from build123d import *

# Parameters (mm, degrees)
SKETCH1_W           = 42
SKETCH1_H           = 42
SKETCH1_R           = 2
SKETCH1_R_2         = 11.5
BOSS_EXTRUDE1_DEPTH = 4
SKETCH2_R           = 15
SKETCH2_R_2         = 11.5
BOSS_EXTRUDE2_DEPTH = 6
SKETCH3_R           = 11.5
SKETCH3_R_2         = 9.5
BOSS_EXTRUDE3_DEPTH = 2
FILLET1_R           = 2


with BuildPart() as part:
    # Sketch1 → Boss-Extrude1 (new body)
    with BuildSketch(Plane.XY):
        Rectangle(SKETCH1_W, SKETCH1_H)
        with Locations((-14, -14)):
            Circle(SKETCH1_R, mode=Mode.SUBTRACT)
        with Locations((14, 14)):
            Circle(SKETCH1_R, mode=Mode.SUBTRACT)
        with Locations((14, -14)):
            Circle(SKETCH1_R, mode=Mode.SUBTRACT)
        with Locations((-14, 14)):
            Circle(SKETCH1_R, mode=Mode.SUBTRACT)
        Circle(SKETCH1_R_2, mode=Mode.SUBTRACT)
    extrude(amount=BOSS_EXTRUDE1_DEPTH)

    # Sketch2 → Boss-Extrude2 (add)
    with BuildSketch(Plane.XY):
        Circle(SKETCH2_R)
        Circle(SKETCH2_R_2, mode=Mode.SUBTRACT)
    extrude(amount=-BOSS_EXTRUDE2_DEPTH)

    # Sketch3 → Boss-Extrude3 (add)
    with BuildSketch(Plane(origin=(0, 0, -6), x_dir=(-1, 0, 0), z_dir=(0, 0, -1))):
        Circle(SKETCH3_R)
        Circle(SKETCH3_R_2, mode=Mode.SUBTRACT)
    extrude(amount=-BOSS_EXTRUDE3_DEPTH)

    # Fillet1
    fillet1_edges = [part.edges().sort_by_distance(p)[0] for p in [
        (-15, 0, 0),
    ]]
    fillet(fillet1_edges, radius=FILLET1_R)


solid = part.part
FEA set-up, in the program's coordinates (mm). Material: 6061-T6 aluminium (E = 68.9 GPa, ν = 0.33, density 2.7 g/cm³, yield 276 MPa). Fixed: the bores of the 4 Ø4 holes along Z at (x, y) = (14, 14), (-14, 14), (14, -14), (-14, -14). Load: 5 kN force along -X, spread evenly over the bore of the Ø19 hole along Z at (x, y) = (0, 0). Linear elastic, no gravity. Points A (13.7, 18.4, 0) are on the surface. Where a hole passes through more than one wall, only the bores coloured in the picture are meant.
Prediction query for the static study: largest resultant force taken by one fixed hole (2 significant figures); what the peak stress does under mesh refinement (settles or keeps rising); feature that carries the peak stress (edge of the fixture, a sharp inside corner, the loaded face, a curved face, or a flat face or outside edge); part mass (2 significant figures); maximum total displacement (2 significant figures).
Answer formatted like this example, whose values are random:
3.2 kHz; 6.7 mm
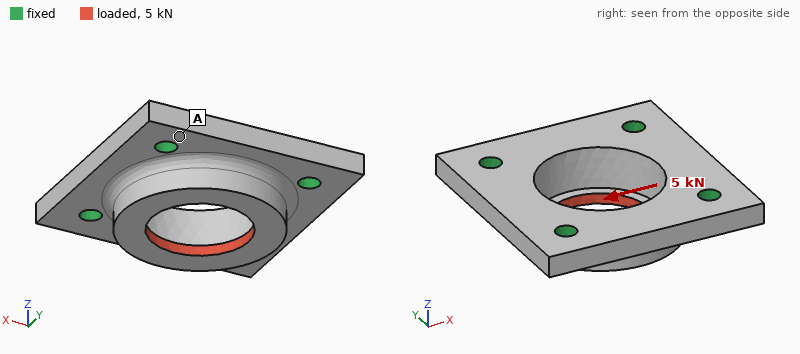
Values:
1.4 kN; keeps rising; edge of the fixture; 20 g; 28 µm
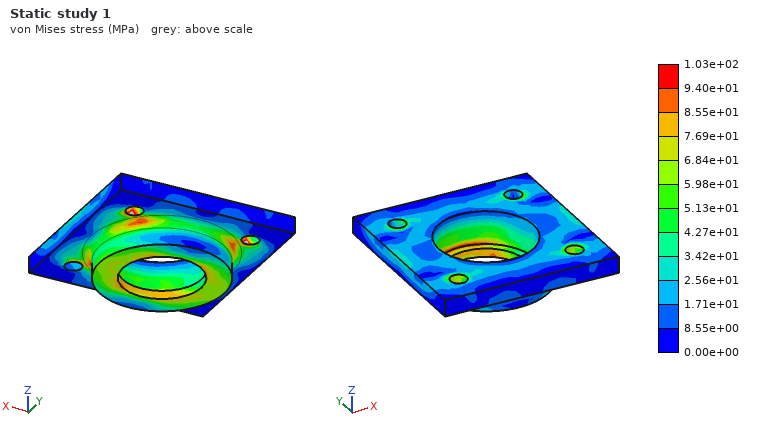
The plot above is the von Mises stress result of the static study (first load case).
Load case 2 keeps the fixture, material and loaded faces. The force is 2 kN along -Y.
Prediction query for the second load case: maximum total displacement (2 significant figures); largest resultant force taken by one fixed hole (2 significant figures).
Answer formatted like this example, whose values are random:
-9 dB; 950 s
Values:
11 µm; 560 N
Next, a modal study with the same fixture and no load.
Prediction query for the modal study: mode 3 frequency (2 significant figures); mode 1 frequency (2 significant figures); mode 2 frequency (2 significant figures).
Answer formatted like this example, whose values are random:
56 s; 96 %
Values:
29 kHz; 27 kHz; 28 kHz
